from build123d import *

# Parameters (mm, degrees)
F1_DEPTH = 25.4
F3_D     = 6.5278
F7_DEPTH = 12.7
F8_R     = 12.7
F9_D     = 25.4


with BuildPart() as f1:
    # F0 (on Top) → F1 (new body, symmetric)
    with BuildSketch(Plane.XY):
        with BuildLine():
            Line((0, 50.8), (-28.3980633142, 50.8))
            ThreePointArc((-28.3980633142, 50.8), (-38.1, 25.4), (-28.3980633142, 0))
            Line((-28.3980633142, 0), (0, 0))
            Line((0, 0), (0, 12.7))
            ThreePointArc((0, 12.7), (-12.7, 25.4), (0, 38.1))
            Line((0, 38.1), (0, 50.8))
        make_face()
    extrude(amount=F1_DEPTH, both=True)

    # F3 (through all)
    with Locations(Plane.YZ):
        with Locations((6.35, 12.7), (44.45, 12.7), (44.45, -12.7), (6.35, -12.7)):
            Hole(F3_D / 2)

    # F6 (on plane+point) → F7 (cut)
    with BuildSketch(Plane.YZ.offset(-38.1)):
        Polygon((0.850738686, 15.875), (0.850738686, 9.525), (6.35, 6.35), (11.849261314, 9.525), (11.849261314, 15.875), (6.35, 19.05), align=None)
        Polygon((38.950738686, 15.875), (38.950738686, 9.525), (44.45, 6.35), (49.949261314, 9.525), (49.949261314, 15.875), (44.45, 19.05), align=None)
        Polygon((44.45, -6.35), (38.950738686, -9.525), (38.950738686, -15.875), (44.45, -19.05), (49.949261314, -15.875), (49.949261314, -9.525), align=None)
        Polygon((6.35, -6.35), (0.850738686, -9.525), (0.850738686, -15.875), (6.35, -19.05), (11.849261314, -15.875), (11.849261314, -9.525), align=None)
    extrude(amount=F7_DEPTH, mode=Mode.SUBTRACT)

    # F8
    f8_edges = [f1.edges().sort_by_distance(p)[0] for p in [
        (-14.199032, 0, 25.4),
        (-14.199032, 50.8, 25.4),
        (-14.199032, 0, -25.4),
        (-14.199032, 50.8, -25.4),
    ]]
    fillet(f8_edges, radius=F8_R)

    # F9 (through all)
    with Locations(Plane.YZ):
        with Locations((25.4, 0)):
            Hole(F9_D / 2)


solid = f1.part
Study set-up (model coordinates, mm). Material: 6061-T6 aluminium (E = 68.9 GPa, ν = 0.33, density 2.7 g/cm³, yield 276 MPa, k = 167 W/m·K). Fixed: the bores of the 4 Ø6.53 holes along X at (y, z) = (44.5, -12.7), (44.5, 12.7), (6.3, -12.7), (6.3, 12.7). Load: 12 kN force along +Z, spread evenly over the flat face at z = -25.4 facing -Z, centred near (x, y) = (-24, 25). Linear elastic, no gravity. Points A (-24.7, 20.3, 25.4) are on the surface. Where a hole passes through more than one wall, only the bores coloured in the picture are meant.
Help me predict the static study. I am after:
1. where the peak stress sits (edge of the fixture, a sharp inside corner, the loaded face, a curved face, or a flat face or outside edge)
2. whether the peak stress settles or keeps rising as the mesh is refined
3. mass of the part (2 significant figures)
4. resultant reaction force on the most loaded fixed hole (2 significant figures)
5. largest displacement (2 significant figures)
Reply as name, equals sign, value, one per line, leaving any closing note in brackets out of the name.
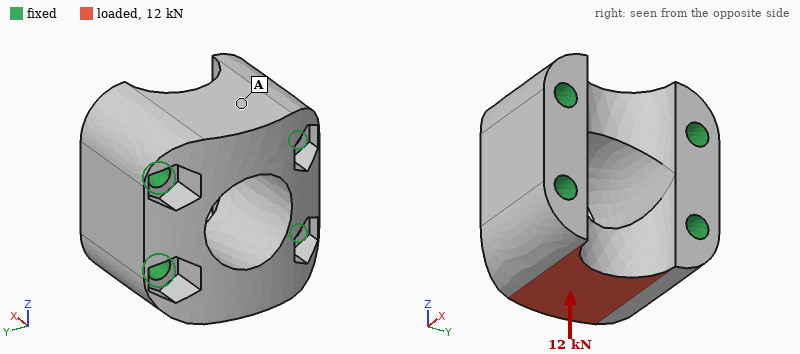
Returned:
where the peak stress sits = edge of the fixture
whether the peak stress settles or keeps rising as the mesh is refined = keeps rising
mass of the part = 140 g
resultant reaction force on the most loaded fixed hole = 5.0 kN
largest displacement = 23 µm
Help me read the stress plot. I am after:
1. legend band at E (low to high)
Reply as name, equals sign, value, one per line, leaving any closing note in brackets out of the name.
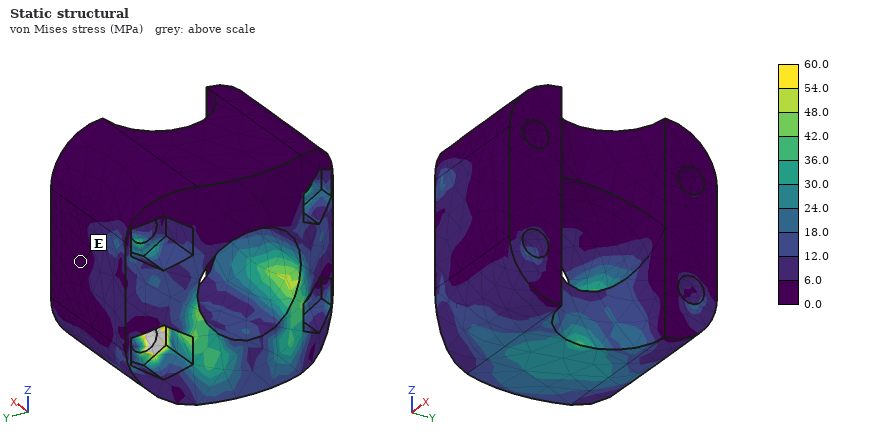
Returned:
legend band at E = 0.0 to 6.0 MPa
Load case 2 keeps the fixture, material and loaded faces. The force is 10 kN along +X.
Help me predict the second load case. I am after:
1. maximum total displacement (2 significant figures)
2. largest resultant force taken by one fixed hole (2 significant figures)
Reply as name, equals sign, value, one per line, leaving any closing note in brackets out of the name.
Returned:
maximum total displacement = 28 µm
largest resultant force taken by one fixed hole = 5.8 kN
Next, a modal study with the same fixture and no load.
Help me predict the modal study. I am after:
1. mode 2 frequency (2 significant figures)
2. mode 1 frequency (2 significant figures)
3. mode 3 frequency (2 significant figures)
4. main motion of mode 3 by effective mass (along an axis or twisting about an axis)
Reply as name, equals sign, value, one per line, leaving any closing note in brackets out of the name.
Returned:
mode 2 frequency = 26 kHz
mode 1 frequency = 25 kHz
mode 3 frequency = 35 kHz
main motion of mode 3 by effective mass = along Y
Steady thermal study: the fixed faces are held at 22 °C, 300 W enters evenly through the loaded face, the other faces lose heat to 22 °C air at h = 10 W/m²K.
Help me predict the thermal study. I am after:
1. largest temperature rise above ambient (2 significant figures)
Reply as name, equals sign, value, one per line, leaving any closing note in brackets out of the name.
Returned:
largest temperature rise above ambient = 52 K
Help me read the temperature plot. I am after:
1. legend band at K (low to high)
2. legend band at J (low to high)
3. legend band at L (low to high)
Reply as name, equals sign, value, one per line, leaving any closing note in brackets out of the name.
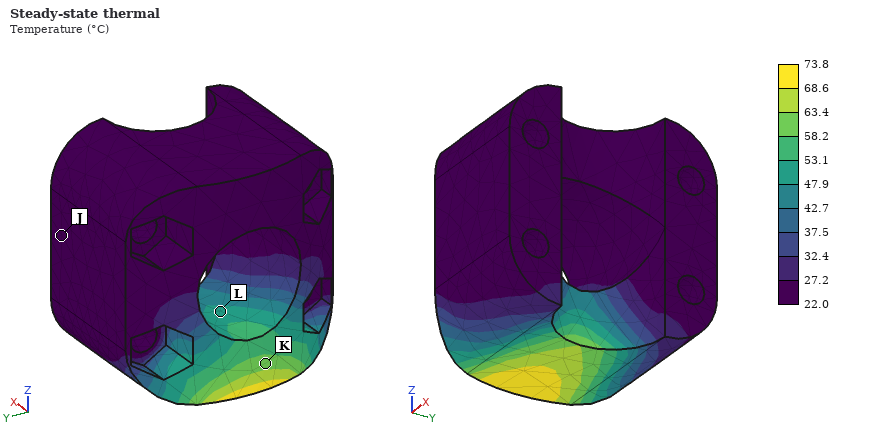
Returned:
legend band at K = 58.2 to 63.4 °C
legend band at J = 22.0 to 27.2 °C
legend band at L = 47.9 to 53.1 °C
